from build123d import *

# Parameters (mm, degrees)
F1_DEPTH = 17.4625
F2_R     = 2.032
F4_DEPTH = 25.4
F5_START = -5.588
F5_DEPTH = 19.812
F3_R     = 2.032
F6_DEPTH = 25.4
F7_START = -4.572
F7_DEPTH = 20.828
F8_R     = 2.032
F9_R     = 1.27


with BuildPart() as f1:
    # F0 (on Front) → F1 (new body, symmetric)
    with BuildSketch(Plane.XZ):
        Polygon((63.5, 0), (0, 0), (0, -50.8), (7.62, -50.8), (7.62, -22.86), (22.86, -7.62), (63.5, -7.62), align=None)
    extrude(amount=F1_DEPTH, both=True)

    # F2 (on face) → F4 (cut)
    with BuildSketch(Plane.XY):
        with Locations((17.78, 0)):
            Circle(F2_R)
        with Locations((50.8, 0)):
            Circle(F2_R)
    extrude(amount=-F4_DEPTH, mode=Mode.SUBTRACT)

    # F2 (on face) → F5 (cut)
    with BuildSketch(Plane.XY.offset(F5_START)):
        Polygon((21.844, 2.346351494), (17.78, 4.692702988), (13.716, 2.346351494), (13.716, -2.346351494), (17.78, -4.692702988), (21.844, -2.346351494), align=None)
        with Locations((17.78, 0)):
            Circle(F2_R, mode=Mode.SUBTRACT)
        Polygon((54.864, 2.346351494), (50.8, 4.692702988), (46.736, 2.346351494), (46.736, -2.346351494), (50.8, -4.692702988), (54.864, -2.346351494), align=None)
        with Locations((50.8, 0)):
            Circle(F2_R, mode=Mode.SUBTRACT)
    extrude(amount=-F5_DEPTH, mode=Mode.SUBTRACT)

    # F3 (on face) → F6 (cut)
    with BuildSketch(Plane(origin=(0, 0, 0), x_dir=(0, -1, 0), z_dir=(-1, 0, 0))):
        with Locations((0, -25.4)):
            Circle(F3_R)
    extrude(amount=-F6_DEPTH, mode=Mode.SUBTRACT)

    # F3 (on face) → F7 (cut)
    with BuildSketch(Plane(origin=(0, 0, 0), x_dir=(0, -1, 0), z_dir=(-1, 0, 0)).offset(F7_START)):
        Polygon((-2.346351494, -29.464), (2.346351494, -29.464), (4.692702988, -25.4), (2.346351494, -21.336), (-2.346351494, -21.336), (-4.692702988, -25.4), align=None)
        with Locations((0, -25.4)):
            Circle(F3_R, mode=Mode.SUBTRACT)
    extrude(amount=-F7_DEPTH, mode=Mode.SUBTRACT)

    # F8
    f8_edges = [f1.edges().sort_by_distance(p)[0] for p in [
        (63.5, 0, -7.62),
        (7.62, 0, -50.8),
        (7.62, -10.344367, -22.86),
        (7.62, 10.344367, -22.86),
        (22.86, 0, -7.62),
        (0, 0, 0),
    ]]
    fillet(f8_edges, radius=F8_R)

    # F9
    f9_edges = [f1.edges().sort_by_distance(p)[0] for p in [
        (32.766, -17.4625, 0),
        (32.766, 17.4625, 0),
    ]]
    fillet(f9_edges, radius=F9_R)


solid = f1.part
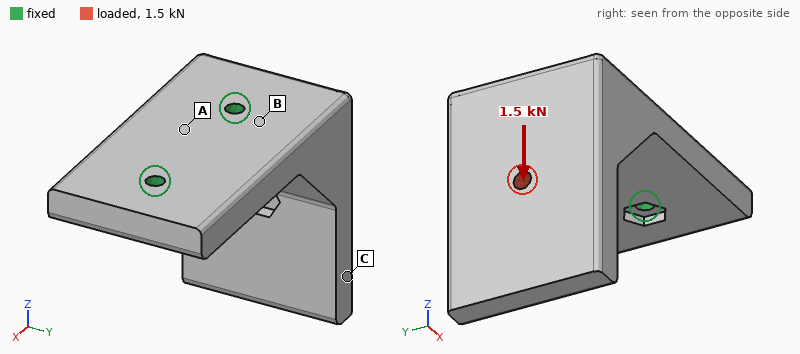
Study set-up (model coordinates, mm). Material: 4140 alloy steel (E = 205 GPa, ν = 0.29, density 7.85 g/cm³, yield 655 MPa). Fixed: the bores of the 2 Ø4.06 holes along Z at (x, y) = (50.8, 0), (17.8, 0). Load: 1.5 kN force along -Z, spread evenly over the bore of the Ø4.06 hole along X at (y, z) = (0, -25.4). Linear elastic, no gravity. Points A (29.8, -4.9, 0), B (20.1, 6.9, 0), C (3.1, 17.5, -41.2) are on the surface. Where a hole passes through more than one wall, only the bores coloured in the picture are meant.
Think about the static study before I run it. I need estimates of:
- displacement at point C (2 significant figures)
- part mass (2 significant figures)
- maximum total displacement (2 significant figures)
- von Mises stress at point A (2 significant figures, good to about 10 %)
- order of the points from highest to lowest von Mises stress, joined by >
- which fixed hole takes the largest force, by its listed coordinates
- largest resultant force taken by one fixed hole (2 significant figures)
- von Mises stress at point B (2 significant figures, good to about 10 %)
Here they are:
26 µm
250 g
34 µm
15 MPa
B > A > C
(17.8, 0)
2.0 kN
28 MPa
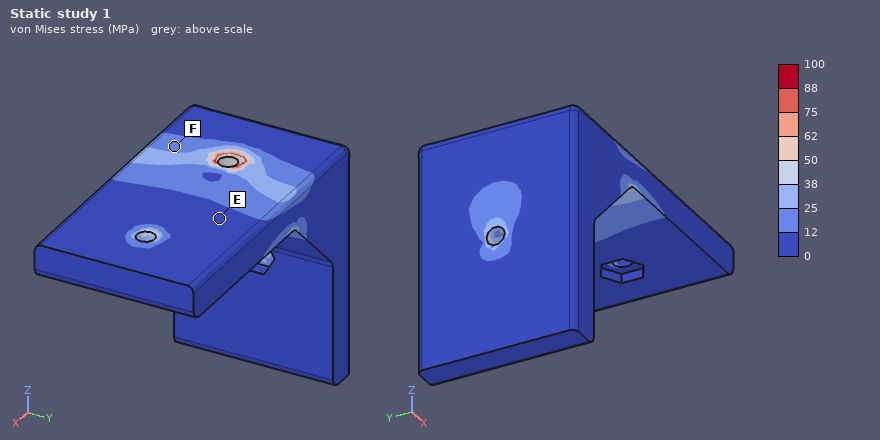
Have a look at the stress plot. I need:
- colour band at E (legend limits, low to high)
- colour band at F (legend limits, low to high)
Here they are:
0 to 12 MPa
12 to 25 MPa
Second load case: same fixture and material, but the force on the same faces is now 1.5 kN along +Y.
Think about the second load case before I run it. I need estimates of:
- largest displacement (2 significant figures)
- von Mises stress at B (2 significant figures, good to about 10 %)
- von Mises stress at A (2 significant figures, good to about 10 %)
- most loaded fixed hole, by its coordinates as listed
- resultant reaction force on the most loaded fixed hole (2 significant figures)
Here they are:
65 µm
30 MPa
27 MPa
(17.8, 0)
2.1 kN
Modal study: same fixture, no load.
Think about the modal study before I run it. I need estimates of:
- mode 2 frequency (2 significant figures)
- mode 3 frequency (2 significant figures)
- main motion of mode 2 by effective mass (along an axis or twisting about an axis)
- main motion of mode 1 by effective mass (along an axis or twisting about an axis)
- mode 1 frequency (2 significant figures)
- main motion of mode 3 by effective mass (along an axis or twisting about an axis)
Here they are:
2800 Hz
8800 Hz
along X
along Y
2600 Hz
along Z
